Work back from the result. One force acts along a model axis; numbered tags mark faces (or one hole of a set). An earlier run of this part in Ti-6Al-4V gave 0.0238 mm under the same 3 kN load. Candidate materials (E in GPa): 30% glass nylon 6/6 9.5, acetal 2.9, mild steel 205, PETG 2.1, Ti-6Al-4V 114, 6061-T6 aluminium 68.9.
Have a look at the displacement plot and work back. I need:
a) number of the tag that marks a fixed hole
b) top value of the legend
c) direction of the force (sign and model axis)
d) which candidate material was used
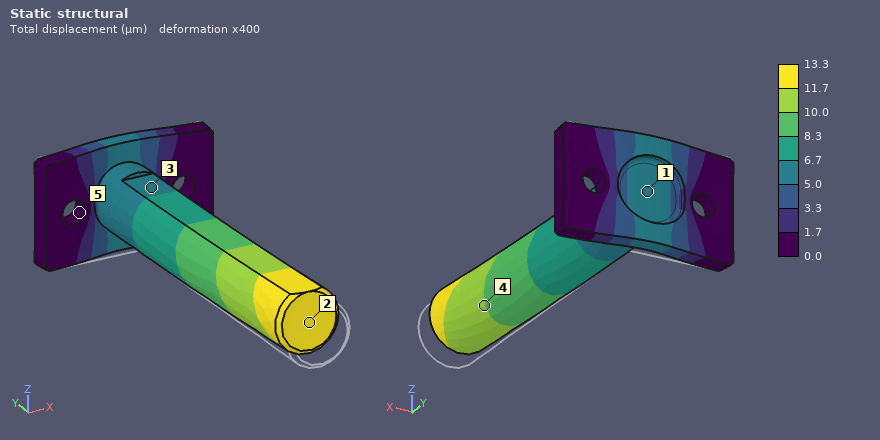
5
13.3 µm
+Y
mild steel
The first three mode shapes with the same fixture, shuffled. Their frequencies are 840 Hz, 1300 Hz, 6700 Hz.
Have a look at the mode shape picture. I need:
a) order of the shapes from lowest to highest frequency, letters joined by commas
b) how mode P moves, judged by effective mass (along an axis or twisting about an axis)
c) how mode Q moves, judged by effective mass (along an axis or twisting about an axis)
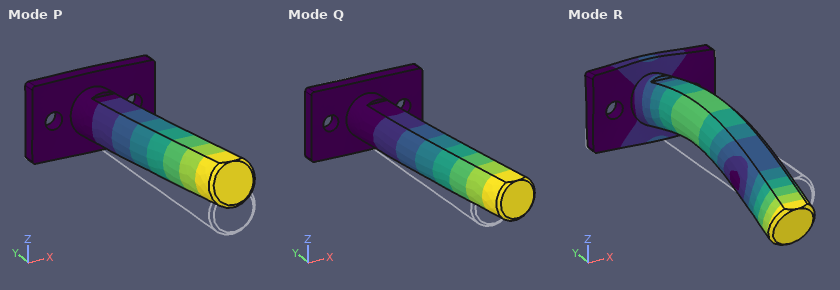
P, Q, R
along Z
along X
